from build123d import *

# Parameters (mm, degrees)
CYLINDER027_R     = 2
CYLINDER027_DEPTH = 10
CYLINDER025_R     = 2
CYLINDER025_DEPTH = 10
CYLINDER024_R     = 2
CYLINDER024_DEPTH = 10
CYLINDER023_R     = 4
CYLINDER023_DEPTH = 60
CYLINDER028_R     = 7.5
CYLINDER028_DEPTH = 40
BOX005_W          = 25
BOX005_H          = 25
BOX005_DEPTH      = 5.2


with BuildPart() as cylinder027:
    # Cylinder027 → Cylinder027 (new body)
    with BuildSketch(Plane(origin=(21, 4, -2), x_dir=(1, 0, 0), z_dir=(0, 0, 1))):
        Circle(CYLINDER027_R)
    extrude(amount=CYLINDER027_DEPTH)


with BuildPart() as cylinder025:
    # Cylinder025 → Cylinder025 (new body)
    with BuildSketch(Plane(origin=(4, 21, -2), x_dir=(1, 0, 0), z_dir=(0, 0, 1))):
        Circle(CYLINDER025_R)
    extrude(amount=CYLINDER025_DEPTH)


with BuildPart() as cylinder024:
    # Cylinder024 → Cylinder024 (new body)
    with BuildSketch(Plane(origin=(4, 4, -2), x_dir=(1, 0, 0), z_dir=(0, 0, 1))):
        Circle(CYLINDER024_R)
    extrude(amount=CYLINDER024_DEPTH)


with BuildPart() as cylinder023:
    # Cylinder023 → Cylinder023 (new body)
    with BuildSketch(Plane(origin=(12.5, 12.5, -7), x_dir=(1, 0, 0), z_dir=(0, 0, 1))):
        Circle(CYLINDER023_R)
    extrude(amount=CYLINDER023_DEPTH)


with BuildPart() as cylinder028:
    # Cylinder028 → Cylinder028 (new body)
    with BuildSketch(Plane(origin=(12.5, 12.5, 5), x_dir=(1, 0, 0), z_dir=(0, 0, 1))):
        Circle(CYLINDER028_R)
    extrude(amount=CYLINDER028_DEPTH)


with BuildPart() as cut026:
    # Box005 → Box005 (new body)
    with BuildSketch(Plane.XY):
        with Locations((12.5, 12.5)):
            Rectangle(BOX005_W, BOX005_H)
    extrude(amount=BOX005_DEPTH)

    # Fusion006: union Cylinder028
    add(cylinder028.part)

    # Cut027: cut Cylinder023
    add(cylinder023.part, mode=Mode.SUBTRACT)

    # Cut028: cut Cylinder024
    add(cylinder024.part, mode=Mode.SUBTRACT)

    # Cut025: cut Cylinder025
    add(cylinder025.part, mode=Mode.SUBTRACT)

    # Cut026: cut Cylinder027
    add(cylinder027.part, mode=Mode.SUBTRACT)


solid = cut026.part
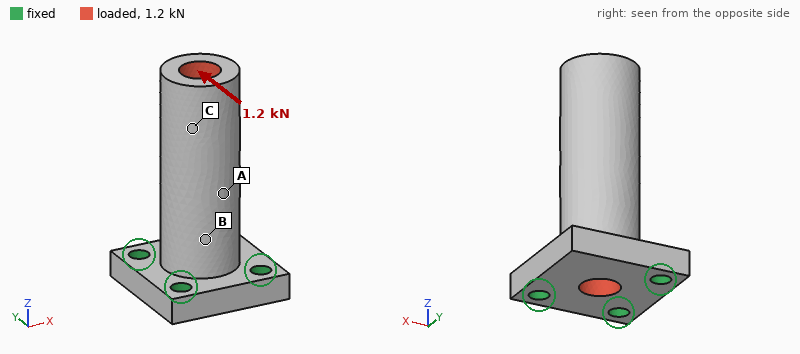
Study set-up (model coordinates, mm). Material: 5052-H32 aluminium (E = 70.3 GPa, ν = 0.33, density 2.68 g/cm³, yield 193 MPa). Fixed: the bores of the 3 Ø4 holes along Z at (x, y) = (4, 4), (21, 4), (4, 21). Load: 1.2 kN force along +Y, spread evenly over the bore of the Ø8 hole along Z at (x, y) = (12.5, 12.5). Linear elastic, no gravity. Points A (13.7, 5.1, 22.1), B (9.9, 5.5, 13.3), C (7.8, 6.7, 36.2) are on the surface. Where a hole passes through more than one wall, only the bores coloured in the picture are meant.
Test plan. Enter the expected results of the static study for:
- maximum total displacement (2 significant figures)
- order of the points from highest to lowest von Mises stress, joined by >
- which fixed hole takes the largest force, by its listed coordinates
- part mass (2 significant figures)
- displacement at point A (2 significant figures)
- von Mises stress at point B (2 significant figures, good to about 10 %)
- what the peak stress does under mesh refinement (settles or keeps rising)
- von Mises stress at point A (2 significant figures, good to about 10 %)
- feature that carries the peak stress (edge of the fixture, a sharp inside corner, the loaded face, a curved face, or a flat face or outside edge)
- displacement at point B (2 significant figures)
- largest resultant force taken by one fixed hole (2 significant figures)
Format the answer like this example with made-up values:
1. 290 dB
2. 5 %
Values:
1. 0.13 mm
2. B > A > C
3. (4, 21)
4. 21 g
5. 0.053 mm
6. 41 MPa
7. keeps rising
8. 23 MPa
9. edge of the fixture
10. 0.027 mm
11. 1.4 kN
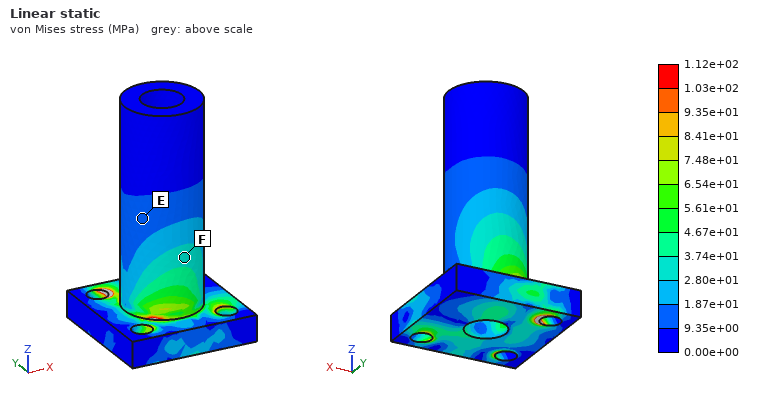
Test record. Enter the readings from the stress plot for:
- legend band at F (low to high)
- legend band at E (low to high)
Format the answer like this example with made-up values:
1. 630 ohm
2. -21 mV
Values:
1. 2.80e+01 to 3.74e+01 MPa
2. 9.35e+00 to 1.87e+01 MPa
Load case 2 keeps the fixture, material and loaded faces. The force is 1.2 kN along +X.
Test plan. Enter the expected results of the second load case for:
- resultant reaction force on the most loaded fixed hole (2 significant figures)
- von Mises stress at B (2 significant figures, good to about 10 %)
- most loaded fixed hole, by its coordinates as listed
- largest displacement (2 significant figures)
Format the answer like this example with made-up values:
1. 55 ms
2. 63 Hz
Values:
1. 1.4 kN
2. 22 MPa
3. (21, 4)
4. 0.13 mm
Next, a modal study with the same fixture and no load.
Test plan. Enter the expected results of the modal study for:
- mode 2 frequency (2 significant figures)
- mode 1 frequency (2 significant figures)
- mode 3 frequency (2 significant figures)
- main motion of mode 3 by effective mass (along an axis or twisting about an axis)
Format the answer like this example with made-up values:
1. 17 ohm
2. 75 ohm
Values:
1. 5400 Hz
2. 4400 Hz
3. 19 kHz
4. twisting about Z
